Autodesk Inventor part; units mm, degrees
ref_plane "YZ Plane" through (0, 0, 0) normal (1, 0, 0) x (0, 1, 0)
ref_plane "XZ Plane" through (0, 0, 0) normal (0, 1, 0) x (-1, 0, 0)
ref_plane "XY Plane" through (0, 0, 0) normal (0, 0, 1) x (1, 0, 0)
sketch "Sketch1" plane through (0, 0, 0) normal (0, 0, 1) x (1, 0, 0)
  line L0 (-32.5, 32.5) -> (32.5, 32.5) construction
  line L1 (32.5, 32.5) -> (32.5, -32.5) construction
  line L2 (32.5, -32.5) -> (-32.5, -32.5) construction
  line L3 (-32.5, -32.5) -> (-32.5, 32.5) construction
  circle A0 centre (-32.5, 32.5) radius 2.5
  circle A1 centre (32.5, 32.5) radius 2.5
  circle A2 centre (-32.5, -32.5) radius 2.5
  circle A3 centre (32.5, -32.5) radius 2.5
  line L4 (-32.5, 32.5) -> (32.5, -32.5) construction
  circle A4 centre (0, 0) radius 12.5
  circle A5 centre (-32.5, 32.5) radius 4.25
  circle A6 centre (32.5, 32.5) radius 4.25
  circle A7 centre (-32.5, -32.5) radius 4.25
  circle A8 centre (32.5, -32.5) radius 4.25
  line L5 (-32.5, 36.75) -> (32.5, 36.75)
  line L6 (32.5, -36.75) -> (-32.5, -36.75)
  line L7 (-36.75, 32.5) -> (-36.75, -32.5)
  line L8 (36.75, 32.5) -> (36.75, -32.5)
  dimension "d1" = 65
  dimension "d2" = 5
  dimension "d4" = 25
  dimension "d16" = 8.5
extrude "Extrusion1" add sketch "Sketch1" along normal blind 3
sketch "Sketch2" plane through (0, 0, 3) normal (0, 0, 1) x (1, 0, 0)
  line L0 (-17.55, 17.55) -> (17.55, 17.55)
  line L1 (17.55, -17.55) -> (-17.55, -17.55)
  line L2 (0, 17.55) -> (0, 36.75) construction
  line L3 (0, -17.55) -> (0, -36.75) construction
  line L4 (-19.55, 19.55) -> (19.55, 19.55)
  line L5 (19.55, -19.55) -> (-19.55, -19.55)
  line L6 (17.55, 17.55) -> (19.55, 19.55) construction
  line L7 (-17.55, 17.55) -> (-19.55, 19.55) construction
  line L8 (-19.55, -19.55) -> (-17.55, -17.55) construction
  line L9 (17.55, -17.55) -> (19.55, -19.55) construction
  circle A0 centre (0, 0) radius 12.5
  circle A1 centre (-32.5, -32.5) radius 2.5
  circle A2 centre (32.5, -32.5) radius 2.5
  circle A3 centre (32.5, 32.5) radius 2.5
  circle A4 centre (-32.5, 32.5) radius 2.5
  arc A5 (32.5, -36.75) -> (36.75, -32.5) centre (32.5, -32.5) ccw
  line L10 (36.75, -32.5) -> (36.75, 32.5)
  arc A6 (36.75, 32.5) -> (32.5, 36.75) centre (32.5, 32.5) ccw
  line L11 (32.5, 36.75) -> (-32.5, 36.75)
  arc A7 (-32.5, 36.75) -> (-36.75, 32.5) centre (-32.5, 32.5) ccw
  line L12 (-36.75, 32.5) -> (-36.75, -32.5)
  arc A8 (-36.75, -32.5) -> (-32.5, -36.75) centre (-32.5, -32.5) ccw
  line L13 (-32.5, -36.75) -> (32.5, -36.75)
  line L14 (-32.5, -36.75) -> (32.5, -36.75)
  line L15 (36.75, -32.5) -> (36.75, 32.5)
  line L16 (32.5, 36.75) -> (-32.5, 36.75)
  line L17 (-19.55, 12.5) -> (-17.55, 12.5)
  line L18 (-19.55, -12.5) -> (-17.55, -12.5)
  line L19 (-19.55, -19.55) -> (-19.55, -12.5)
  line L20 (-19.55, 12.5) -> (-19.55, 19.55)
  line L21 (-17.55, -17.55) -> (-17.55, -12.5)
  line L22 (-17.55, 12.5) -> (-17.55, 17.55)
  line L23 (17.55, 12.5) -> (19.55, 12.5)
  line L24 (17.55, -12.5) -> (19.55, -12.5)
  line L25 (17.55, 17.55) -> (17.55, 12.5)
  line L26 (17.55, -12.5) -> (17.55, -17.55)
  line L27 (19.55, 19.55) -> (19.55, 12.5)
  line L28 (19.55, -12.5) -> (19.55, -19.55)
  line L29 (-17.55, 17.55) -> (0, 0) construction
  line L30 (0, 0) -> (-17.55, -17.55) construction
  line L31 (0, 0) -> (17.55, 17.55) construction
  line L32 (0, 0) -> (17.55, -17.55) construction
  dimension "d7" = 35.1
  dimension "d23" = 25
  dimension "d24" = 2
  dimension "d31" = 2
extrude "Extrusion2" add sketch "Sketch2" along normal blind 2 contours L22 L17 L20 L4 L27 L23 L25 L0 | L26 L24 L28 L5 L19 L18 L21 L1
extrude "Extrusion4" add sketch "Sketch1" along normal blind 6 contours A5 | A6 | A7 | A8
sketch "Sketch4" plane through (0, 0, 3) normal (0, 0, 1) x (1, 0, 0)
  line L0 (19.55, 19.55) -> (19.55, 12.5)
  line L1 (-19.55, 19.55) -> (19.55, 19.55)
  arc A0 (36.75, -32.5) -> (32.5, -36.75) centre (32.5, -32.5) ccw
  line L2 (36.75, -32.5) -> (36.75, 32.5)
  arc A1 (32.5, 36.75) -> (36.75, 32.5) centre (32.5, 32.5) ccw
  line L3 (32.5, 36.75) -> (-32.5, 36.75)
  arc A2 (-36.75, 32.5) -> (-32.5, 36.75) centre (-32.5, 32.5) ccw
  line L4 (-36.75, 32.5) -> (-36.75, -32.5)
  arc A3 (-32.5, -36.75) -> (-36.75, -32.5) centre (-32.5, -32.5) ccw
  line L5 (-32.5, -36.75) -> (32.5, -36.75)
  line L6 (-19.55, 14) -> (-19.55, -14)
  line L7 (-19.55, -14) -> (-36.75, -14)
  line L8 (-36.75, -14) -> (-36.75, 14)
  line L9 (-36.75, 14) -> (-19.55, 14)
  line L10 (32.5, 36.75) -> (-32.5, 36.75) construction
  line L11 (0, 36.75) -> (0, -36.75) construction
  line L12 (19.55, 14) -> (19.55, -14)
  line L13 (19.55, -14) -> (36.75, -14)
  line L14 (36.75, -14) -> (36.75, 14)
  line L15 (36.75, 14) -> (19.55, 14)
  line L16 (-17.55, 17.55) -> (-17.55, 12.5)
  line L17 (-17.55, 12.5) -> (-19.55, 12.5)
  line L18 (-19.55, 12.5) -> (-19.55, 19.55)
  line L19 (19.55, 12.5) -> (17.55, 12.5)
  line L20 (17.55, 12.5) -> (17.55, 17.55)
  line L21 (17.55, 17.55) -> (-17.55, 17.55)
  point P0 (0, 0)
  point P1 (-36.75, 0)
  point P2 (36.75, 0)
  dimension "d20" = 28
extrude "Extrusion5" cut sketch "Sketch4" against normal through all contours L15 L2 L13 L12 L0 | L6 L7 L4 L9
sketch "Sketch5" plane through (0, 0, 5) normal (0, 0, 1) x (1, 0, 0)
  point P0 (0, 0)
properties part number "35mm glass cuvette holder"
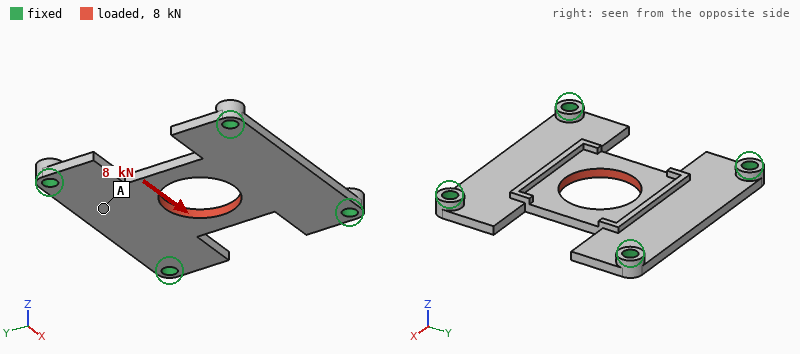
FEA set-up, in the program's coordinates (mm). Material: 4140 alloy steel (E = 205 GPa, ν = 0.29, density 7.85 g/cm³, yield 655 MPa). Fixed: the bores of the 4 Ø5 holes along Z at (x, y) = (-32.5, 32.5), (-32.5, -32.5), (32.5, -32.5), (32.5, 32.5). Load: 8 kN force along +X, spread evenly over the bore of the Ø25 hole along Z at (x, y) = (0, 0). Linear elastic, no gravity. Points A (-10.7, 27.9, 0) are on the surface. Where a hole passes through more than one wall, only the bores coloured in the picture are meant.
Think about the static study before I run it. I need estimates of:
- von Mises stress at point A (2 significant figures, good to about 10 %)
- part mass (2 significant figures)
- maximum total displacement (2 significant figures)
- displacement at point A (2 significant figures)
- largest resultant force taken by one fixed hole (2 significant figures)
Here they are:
26 MPa
97 g
17 µm
3.8 µm
2.3 kN
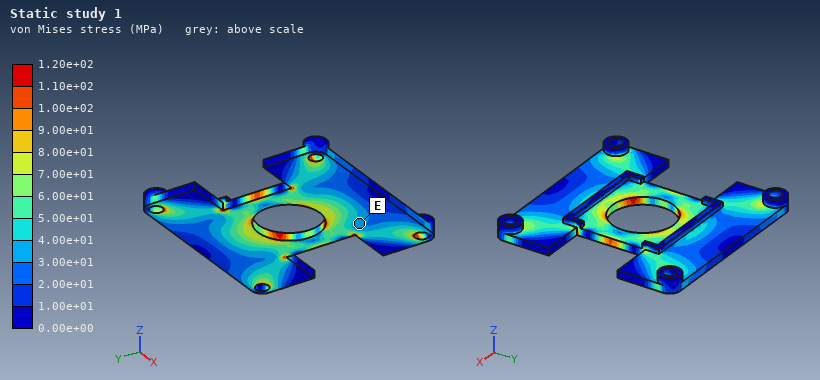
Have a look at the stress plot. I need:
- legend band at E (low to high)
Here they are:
3.00e+01 to 4.00e+01 MPa
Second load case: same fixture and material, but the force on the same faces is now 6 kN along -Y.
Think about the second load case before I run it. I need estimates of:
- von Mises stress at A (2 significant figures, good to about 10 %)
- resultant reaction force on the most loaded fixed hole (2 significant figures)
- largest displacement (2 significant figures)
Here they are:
19 MPa
1.9 kN
13 µm
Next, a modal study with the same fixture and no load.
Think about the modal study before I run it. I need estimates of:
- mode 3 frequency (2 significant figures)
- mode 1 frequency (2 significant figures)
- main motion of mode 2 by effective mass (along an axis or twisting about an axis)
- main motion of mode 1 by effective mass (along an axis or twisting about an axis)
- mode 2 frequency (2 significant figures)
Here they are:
5600 Hz
2800 Hz
twisting about X
along Z
4300 Hz
